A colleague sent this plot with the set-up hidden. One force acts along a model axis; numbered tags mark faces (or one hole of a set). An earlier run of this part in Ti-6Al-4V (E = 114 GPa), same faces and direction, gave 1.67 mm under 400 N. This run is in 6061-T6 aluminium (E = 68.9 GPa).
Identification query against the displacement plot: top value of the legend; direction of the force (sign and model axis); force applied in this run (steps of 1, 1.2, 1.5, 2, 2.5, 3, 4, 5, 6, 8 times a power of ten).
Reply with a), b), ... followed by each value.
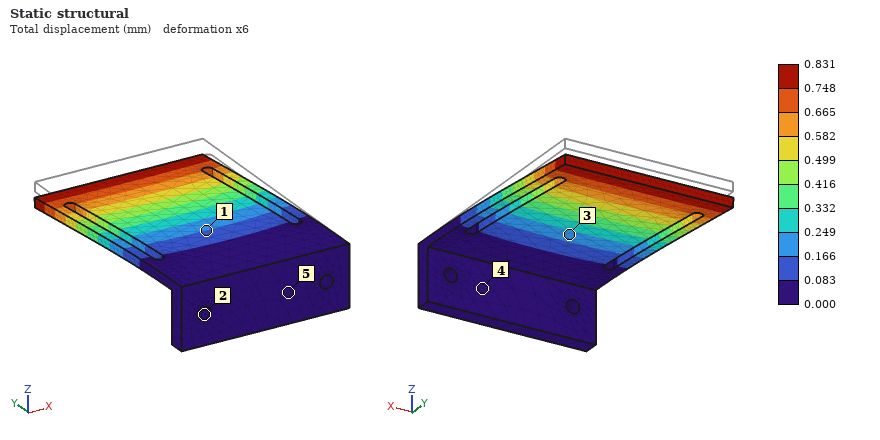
a) 0.831 mm
b) -Z
c) 120 N
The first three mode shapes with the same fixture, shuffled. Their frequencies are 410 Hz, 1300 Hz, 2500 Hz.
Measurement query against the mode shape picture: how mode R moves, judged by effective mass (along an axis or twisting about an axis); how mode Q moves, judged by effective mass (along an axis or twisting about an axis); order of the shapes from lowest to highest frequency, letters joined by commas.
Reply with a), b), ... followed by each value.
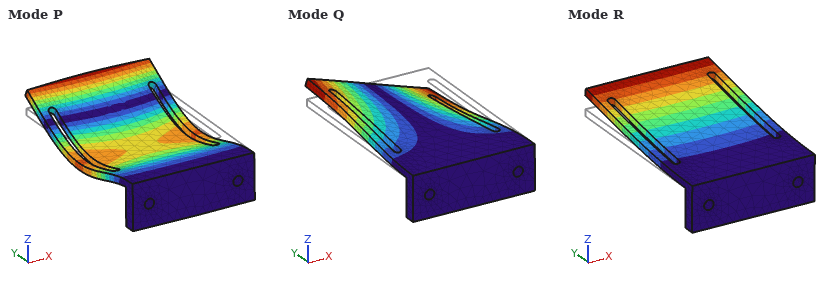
a) along Z
b) twisting about Y
c) R, Q, P
